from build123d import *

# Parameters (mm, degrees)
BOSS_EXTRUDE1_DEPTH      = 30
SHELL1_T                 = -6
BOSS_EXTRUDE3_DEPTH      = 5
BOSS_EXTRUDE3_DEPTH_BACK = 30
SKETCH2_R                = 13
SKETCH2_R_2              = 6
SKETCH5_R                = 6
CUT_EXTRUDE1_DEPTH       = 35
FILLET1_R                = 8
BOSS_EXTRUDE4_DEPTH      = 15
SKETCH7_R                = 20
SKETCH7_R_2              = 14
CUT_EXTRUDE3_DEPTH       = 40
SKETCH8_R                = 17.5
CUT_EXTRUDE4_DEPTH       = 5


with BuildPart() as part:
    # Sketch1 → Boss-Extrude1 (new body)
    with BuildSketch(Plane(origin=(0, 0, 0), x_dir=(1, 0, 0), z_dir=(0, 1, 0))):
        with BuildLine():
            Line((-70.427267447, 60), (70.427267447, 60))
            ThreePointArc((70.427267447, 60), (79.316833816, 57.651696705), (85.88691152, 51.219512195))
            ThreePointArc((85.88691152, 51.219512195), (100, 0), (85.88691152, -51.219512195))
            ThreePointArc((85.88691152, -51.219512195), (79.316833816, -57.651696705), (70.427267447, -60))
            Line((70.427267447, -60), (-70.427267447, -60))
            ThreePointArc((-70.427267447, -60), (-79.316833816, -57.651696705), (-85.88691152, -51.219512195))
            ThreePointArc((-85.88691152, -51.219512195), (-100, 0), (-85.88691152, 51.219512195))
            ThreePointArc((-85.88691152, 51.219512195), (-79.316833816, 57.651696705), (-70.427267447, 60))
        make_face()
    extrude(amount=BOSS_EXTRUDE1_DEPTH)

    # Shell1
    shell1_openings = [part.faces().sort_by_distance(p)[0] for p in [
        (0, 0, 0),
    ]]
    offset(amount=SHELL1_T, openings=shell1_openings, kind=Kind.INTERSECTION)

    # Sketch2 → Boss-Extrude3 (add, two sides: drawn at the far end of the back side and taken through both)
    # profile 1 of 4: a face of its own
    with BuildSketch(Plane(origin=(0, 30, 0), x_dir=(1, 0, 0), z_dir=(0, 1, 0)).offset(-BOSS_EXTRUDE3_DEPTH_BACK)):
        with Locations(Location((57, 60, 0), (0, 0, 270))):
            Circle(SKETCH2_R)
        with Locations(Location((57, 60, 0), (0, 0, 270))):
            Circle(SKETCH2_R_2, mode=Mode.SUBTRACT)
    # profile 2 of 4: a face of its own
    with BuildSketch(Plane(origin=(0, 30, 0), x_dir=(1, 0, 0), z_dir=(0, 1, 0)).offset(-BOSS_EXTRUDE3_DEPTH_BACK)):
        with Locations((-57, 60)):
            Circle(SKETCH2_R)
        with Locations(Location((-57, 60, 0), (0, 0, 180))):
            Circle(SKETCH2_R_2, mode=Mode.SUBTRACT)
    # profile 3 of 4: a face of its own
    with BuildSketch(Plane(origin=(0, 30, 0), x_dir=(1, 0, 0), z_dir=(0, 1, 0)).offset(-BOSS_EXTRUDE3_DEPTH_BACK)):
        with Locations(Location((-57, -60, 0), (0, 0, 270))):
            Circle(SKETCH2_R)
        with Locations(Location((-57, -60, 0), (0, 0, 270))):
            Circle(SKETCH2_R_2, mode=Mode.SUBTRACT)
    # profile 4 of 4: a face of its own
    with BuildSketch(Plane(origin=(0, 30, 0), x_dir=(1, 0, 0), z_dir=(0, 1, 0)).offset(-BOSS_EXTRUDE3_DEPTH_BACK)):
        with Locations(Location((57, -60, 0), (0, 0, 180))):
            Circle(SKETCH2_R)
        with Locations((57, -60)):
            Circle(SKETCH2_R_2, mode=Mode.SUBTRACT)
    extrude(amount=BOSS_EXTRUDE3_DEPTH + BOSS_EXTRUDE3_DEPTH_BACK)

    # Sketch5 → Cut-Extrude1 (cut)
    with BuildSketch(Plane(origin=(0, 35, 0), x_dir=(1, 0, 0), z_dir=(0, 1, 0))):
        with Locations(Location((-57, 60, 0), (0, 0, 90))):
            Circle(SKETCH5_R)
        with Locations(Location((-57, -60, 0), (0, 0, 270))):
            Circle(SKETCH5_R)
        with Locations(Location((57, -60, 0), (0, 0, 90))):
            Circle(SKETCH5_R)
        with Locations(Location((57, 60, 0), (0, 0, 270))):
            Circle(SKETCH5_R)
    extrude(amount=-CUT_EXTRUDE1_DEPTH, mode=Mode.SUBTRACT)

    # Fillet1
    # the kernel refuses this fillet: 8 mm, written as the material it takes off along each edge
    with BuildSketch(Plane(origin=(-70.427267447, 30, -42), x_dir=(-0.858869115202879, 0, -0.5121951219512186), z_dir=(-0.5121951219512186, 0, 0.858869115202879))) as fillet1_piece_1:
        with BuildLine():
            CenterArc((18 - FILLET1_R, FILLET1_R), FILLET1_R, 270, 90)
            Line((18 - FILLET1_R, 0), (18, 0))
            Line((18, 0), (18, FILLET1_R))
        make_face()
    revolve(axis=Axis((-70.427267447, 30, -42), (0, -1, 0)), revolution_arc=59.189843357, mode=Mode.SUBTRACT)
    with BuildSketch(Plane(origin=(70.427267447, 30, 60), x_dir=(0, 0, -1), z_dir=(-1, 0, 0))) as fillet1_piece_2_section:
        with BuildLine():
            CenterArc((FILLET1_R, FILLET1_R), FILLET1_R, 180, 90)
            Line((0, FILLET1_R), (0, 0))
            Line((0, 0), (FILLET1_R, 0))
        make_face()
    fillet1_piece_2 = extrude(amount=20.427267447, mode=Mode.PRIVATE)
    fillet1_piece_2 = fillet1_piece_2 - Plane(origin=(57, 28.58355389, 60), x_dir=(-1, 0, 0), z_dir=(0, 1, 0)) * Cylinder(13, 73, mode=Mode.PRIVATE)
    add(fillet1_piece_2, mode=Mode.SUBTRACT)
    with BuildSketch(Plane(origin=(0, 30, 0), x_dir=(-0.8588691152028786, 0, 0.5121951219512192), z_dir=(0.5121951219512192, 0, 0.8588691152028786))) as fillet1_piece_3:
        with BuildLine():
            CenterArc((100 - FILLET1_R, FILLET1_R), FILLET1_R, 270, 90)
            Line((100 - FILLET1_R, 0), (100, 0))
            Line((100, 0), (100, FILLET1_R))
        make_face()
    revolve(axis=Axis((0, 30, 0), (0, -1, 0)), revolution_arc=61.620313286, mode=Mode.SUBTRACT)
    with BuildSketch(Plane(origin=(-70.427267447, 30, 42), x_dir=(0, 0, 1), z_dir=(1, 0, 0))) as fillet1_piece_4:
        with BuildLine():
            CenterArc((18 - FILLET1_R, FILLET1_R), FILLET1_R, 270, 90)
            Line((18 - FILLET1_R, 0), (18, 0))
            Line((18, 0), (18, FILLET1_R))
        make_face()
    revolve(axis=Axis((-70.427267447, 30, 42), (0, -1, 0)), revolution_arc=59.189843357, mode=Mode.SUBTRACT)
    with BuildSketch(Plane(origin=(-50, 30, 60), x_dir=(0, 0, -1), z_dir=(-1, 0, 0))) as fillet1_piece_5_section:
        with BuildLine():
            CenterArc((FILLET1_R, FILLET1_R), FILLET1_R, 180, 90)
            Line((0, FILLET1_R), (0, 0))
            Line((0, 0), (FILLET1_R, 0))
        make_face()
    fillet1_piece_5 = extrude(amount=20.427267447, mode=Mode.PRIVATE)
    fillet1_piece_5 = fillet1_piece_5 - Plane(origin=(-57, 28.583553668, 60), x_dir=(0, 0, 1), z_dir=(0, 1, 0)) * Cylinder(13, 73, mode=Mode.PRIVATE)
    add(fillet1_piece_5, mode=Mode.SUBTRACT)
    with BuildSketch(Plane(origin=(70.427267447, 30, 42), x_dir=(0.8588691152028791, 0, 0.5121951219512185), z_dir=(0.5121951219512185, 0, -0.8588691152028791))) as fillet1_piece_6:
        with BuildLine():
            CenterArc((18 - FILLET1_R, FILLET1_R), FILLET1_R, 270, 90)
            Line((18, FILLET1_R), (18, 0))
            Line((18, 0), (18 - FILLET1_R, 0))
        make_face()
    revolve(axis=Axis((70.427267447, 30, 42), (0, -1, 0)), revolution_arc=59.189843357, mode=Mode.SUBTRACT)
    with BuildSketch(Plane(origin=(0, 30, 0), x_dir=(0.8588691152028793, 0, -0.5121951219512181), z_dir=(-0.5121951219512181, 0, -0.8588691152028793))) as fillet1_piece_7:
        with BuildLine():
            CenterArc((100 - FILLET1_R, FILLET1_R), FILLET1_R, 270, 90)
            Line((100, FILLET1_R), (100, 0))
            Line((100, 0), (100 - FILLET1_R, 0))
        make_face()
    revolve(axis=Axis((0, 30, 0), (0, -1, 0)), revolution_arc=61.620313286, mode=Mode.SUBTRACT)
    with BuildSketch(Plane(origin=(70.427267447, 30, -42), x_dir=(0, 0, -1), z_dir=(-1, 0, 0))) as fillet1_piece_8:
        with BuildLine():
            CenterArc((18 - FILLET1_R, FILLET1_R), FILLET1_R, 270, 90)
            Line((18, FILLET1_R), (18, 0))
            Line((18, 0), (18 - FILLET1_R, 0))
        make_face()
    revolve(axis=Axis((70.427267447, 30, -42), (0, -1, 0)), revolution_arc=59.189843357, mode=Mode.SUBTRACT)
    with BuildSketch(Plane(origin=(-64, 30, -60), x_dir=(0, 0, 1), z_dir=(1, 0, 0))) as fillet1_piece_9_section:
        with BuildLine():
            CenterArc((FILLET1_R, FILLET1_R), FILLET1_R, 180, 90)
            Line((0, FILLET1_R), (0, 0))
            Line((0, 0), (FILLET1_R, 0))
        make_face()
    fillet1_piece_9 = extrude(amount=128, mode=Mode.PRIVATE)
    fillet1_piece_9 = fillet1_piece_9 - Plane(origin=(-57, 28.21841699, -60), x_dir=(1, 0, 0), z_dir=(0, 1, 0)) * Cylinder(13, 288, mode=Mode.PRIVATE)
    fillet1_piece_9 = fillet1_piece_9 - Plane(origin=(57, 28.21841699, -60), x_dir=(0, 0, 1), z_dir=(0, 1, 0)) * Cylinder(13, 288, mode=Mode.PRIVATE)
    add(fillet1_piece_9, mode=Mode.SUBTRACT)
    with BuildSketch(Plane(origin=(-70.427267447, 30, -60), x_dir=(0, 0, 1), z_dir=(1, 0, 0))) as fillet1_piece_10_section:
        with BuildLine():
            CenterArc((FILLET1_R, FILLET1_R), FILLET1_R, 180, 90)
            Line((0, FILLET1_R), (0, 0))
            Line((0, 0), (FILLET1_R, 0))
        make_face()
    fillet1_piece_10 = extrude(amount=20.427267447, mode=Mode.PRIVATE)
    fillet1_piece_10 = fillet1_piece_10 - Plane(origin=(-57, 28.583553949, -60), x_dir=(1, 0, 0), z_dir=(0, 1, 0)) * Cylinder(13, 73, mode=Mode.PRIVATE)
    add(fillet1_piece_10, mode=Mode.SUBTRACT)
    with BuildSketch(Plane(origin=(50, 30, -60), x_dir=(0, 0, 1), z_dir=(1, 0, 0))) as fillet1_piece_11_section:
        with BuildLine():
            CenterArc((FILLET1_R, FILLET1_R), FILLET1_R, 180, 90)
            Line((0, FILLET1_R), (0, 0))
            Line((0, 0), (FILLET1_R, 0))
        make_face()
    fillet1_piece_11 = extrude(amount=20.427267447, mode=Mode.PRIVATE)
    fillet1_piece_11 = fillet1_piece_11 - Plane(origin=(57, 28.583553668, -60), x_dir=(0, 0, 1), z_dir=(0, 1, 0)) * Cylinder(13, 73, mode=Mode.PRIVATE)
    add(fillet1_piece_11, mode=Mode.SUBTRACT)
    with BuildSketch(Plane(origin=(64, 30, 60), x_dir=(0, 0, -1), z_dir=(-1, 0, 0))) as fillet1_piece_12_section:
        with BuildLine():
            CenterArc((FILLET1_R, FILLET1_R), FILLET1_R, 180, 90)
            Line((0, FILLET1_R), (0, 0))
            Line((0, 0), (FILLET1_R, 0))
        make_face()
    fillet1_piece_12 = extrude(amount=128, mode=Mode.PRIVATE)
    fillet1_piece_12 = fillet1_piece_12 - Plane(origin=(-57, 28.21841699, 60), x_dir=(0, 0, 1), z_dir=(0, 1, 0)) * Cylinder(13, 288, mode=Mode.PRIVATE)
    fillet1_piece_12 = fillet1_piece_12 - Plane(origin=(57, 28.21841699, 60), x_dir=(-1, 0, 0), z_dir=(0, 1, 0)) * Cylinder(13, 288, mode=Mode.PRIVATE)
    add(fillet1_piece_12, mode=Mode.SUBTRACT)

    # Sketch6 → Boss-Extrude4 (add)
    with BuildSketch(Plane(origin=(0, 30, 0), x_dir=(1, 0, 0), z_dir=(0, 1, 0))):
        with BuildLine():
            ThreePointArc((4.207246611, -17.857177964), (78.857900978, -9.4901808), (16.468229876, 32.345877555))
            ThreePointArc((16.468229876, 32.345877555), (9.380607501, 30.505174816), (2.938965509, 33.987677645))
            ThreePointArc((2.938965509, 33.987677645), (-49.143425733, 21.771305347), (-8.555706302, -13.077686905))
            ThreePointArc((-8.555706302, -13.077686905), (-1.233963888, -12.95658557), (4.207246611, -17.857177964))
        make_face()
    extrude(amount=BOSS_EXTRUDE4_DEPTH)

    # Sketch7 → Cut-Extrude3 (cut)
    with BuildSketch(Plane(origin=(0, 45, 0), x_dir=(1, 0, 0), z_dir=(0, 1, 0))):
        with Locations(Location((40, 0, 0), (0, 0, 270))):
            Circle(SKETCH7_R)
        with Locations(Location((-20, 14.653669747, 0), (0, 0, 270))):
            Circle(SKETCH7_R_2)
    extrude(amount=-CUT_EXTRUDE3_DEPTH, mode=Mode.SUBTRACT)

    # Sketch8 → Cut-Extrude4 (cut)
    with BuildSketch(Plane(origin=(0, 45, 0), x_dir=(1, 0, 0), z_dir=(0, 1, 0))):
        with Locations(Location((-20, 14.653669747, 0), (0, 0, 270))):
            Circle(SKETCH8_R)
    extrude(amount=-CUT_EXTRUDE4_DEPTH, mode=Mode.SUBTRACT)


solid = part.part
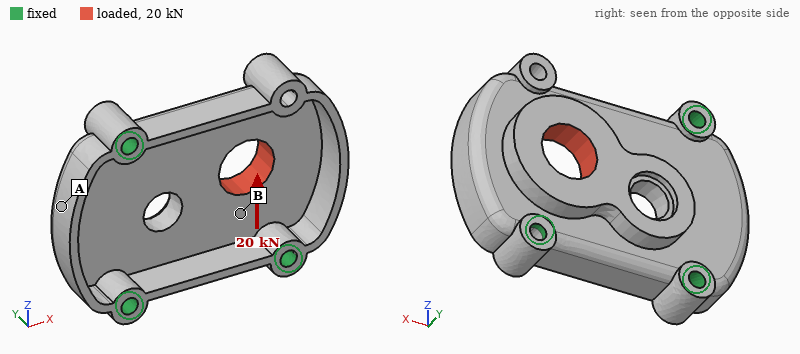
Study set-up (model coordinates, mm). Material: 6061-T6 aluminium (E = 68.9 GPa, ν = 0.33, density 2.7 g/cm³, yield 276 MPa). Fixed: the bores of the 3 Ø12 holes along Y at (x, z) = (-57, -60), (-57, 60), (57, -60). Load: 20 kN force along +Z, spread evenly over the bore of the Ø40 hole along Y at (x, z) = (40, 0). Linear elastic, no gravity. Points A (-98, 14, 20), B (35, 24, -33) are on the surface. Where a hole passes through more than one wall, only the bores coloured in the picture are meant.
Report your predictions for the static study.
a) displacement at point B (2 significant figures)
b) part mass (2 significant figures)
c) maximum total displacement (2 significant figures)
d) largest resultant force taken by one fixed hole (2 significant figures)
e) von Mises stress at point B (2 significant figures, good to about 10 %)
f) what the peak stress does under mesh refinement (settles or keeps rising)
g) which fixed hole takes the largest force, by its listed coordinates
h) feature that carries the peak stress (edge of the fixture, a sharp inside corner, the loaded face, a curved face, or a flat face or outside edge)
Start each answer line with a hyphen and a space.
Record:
- 0.022 mm
- 860 g
- 0.12 mm
- 12 kN
- 27 MPa
- keeps rising
- (57, -60)
- a sharp inside corner
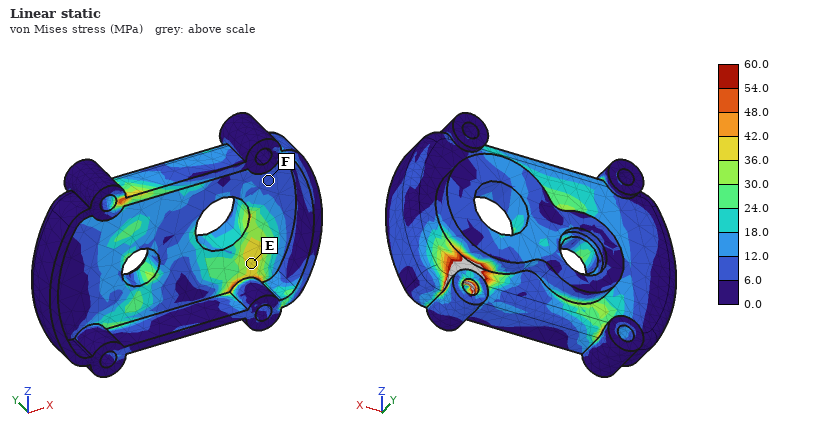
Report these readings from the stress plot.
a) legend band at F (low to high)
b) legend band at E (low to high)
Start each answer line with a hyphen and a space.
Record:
- 6.0 to 12.0 MPa
- 36.0 to 42.0 MPa
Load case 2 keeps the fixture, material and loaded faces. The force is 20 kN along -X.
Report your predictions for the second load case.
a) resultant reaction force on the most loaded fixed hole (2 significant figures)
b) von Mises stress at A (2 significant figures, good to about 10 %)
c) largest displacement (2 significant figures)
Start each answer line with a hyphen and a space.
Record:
- 7.7 kN
- 5.6 MPa
- 0.15 mm
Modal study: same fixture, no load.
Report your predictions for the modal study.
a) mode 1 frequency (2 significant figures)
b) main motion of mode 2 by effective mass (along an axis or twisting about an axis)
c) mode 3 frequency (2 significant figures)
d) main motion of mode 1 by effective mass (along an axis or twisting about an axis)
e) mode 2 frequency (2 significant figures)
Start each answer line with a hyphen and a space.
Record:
- 1200 Hz
- along Y
- 3200 Hz
- along Y
- 2800 Hz
